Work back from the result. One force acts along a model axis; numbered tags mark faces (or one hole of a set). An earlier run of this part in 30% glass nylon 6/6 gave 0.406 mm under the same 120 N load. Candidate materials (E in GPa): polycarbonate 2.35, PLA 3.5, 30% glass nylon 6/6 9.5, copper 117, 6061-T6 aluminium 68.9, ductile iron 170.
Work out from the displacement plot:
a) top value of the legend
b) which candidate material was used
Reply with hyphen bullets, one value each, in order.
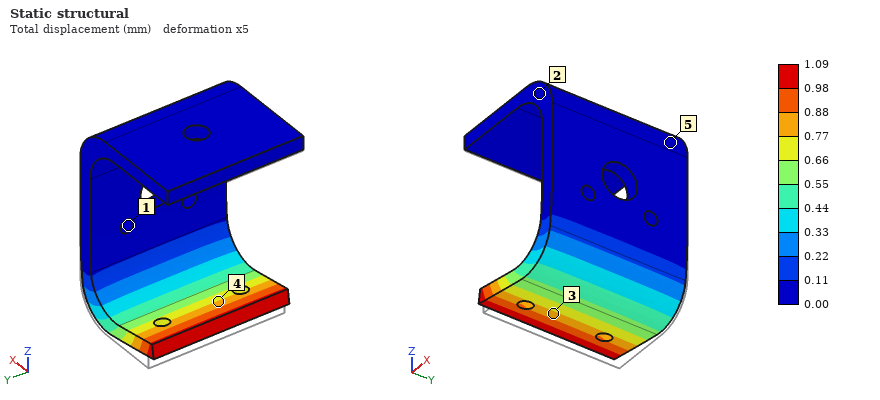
- 1.09 mm
- PLA
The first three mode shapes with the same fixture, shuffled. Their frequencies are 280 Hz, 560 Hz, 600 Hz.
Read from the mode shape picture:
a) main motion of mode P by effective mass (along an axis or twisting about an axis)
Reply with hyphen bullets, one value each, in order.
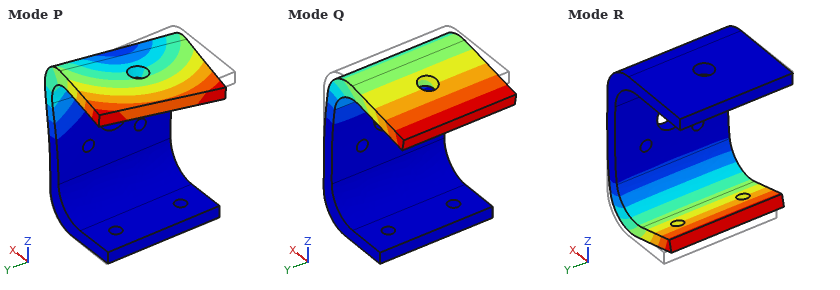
- along Y
